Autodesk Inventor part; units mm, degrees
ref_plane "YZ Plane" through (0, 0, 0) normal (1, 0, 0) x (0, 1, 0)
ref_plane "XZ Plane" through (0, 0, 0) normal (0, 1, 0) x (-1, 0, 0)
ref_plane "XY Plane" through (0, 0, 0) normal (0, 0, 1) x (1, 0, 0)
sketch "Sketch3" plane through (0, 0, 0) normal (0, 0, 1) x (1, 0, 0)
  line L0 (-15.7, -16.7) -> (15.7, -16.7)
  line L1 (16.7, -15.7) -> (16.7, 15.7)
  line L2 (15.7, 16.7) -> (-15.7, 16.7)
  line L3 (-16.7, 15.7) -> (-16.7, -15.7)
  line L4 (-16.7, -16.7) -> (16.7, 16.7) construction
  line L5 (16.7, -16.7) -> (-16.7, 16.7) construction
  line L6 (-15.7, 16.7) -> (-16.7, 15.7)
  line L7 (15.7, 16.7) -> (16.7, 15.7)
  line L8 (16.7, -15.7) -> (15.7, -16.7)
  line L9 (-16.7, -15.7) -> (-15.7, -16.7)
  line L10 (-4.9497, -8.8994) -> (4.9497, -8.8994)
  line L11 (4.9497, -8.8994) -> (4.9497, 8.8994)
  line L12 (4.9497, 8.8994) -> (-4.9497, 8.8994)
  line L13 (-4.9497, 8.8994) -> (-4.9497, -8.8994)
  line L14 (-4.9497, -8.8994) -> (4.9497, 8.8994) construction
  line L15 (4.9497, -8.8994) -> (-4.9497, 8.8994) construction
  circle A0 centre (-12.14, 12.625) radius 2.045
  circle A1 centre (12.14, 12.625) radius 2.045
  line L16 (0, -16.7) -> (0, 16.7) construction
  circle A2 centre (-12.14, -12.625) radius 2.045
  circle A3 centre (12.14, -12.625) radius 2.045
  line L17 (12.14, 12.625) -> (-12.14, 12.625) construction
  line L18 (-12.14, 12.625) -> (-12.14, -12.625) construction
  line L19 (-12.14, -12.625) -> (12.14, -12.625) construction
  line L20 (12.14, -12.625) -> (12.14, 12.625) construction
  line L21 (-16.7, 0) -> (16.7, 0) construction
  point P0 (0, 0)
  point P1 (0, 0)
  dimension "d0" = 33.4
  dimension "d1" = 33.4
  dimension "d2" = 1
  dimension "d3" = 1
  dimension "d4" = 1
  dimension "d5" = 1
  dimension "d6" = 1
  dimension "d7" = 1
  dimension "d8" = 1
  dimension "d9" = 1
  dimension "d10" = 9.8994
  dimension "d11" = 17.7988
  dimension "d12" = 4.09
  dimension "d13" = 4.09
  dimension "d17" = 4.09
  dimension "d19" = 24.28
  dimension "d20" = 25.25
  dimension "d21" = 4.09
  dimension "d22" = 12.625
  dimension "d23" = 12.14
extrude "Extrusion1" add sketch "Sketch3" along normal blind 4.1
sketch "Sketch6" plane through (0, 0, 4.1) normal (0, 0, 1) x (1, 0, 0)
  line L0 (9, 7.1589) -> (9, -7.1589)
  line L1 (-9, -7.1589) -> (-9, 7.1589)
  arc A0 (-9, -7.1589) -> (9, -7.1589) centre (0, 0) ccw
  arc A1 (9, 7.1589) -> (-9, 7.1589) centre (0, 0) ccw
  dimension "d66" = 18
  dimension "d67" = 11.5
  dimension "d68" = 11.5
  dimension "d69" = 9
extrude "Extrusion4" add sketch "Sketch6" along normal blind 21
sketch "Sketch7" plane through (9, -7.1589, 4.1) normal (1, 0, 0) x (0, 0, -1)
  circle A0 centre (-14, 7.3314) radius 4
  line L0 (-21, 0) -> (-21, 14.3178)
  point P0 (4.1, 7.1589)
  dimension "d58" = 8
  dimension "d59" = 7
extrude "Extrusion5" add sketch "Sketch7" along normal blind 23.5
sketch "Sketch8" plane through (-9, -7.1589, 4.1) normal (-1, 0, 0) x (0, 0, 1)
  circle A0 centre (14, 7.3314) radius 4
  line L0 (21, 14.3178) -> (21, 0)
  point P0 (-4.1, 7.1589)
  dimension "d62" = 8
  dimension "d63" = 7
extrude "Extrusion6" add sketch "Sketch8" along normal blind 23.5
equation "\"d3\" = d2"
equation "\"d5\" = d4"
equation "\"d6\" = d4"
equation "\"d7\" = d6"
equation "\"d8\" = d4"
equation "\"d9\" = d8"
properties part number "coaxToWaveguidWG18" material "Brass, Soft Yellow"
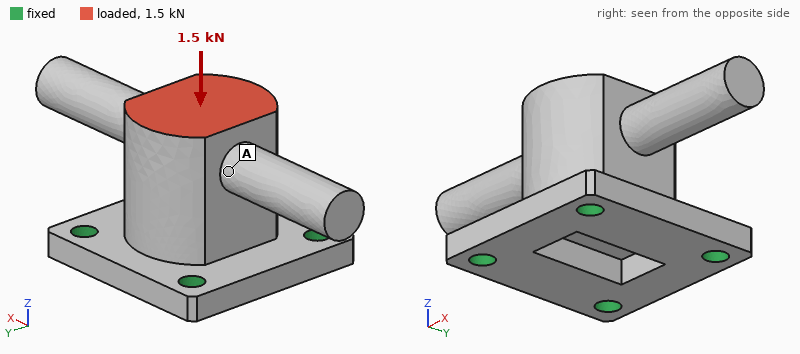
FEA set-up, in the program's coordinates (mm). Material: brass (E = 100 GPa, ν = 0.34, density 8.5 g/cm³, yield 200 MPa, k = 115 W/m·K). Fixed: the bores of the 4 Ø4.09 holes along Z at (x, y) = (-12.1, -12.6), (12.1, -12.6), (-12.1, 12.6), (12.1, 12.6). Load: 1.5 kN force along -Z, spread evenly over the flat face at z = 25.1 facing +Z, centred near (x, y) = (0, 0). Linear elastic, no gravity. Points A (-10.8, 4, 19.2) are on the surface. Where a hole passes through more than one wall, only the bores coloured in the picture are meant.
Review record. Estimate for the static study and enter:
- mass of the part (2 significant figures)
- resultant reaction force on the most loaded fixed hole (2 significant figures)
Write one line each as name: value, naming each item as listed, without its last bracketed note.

mass of the part: 120 g
resultant reaction force on the most loaded fixed hole: 430 N
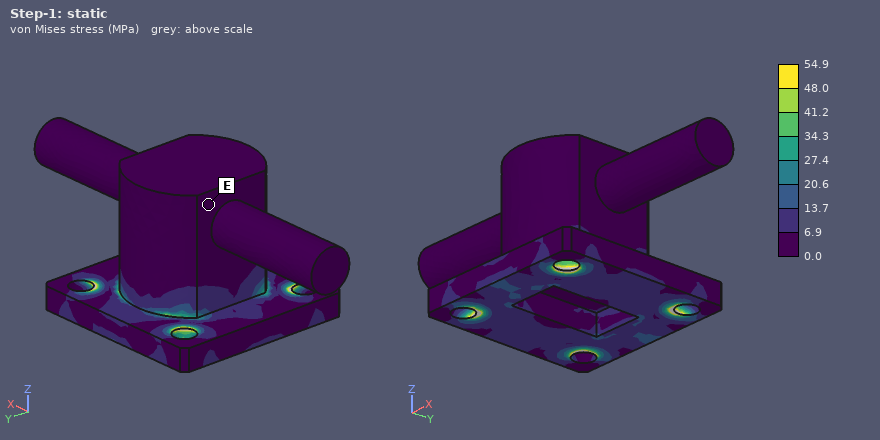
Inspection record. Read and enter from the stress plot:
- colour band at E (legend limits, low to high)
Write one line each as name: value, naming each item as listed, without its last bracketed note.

colour band at E: 0.0 to 6.9 MPa
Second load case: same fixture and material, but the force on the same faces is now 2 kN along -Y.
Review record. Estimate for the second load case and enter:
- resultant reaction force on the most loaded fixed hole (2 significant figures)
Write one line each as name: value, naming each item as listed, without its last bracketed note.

resultant reaction force on the most loaded fixed hole: 1.2 kN
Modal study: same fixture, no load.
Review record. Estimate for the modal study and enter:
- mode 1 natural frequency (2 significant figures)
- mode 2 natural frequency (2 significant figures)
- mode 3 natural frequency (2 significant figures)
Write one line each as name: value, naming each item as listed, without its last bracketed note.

mode 1 natural frequency: 4100 Hz
mode 2 natural frequency: 5100 Hz
mode 3 natural frequency: 5100 Hz
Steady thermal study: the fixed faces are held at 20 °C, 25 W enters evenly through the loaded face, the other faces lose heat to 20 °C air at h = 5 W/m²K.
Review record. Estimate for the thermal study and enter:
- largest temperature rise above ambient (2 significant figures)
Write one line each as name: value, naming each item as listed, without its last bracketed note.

largest temperature rise above ambient: 22 K
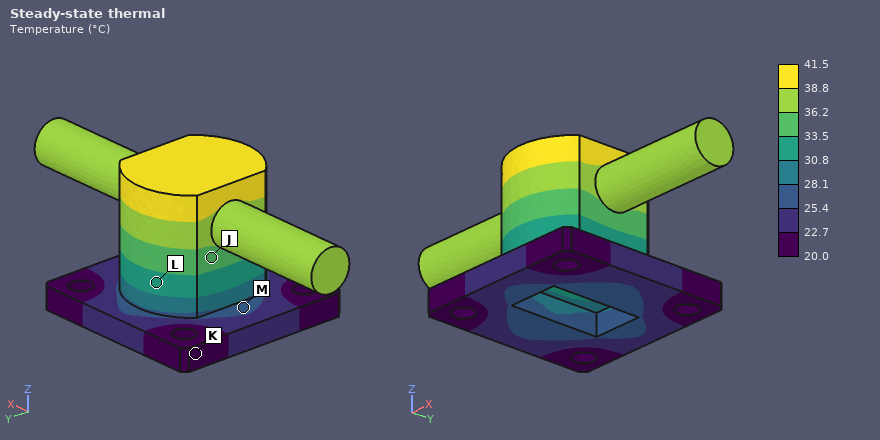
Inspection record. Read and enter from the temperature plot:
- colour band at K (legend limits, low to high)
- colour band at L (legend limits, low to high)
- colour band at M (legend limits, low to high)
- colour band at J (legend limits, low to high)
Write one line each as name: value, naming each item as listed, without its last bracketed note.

colour band at K: 20.0 to 22.7 °C
colour band at L: 30.8 to 33.5 °C
colour band at M: 25.4 to 28.1 °C
colour band at J: 33.5 to 36.2 °C
